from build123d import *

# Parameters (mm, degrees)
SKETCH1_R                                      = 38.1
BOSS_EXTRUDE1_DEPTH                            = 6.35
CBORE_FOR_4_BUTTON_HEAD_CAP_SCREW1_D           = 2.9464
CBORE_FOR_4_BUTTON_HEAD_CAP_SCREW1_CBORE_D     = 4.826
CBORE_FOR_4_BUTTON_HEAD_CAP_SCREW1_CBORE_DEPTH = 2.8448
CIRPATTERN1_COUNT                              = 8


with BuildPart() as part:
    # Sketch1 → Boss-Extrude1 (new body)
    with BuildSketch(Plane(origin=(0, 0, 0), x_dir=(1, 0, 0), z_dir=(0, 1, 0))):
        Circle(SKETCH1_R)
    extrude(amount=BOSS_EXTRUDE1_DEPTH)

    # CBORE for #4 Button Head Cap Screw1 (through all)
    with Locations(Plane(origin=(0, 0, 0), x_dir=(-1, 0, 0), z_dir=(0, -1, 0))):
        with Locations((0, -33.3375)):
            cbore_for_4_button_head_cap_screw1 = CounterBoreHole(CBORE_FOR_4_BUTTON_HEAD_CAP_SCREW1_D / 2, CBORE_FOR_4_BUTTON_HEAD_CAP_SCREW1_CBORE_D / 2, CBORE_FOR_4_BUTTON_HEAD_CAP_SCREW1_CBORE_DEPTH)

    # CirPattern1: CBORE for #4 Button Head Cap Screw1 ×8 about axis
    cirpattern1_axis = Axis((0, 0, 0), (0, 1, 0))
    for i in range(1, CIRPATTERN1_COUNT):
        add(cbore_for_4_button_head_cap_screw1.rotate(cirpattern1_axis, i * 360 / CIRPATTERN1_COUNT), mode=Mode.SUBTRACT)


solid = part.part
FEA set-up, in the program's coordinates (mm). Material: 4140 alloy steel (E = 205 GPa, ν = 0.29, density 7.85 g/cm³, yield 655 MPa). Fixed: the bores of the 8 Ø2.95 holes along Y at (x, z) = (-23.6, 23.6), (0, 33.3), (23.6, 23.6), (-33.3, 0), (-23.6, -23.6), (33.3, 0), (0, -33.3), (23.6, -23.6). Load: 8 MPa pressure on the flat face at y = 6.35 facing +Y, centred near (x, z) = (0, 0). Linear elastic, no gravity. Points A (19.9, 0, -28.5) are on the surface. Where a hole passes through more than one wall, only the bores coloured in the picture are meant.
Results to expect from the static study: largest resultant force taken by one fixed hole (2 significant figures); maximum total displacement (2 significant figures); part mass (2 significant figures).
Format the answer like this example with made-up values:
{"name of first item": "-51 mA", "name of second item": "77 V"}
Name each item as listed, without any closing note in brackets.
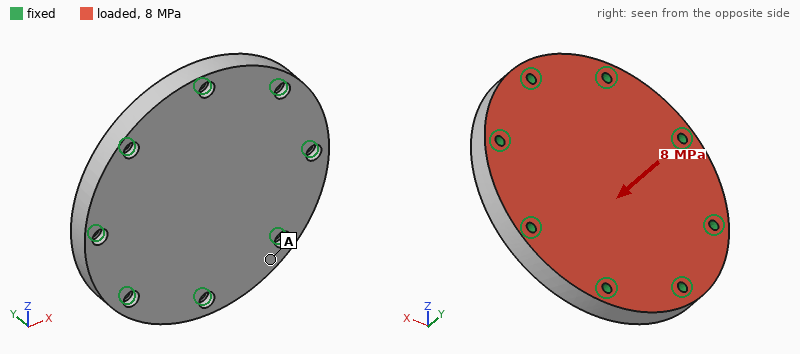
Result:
{"largest resultant force taken by one fixed hole": "5.1 kN", "maximum total displacement": "70 µm", "part mass": "220 g"}
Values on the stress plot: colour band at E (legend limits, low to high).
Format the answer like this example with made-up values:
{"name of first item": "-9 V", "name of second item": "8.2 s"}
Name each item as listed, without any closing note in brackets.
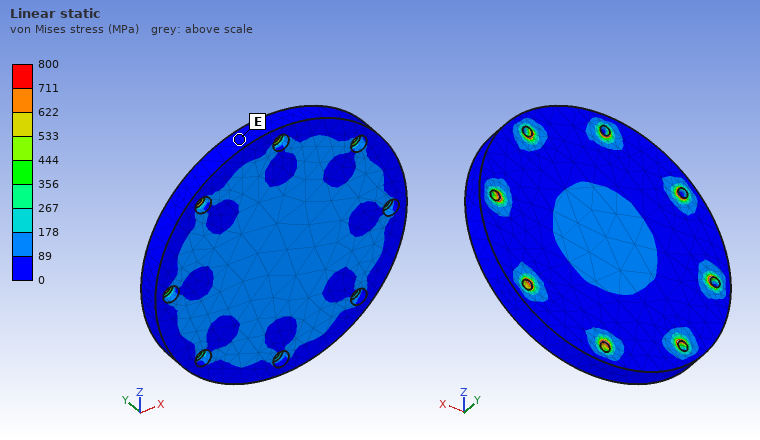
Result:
{"colour band at E": "0 to 89 MPa"}
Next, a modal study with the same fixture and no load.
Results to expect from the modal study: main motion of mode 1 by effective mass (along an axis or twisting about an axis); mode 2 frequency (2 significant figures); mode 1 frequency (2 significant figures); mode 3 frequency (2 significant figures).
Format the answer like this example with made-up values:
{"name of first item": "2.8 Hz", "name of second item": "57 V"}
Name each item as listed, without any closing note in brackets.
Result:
{"main motion of mode 1 by effective mass": "along Y", "mode 2 frequency": "19 kHz", "mode 1 frequency": "9300 Hz", "mode 3 frequency": "19 kHz"}
